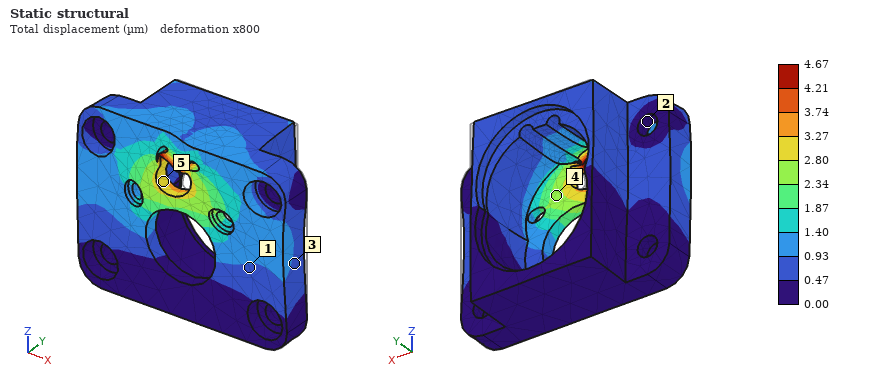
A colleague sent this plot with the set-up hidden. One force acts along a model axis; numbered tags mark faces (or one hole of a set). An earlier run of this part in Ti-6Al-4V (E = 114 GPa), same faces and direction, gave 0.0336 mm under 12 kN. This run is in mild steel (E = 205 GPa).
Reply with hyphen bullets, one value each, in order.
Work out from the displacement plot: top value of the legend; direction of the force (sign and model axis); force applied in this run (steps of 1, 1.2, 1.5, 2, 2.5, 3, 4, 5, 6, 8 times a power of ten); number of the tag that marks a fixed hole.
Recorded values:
- 4.67 µm
- -X
- 3 kN
- 2
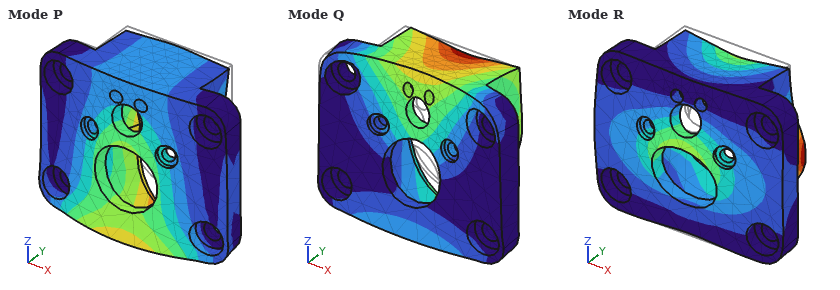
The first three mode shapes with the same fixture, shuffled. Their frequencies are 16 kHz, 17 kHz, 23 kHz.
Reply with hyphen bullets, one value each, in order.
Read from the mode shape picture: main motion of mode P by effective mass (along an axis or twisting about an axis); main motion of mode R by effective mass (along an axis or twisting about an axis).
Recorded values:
- along Y
- along Y
